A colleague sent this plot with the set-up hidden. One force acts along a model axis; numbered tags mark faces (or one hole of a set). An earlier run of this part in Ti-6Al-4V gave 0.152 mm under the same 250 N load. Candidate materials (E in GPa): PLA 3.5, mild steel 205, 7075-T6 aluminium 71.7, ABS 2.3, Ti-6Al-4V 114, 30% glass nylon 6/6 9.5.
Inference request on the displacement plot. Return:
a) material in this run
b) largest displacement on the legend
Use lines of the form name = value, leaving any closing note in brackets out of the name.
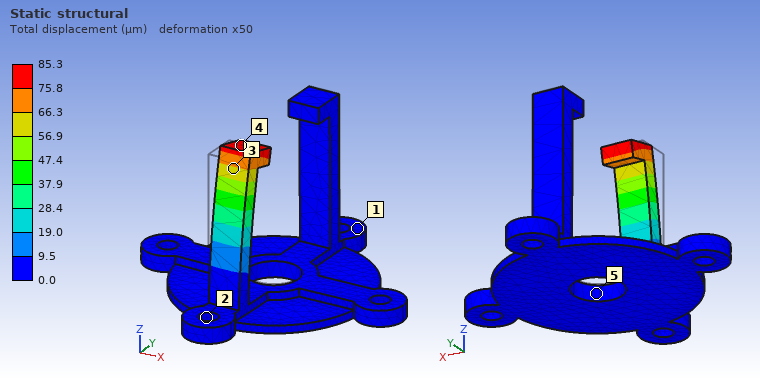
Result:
material in this run = mild steel
largest displacement on the legend = 85.3 µm
